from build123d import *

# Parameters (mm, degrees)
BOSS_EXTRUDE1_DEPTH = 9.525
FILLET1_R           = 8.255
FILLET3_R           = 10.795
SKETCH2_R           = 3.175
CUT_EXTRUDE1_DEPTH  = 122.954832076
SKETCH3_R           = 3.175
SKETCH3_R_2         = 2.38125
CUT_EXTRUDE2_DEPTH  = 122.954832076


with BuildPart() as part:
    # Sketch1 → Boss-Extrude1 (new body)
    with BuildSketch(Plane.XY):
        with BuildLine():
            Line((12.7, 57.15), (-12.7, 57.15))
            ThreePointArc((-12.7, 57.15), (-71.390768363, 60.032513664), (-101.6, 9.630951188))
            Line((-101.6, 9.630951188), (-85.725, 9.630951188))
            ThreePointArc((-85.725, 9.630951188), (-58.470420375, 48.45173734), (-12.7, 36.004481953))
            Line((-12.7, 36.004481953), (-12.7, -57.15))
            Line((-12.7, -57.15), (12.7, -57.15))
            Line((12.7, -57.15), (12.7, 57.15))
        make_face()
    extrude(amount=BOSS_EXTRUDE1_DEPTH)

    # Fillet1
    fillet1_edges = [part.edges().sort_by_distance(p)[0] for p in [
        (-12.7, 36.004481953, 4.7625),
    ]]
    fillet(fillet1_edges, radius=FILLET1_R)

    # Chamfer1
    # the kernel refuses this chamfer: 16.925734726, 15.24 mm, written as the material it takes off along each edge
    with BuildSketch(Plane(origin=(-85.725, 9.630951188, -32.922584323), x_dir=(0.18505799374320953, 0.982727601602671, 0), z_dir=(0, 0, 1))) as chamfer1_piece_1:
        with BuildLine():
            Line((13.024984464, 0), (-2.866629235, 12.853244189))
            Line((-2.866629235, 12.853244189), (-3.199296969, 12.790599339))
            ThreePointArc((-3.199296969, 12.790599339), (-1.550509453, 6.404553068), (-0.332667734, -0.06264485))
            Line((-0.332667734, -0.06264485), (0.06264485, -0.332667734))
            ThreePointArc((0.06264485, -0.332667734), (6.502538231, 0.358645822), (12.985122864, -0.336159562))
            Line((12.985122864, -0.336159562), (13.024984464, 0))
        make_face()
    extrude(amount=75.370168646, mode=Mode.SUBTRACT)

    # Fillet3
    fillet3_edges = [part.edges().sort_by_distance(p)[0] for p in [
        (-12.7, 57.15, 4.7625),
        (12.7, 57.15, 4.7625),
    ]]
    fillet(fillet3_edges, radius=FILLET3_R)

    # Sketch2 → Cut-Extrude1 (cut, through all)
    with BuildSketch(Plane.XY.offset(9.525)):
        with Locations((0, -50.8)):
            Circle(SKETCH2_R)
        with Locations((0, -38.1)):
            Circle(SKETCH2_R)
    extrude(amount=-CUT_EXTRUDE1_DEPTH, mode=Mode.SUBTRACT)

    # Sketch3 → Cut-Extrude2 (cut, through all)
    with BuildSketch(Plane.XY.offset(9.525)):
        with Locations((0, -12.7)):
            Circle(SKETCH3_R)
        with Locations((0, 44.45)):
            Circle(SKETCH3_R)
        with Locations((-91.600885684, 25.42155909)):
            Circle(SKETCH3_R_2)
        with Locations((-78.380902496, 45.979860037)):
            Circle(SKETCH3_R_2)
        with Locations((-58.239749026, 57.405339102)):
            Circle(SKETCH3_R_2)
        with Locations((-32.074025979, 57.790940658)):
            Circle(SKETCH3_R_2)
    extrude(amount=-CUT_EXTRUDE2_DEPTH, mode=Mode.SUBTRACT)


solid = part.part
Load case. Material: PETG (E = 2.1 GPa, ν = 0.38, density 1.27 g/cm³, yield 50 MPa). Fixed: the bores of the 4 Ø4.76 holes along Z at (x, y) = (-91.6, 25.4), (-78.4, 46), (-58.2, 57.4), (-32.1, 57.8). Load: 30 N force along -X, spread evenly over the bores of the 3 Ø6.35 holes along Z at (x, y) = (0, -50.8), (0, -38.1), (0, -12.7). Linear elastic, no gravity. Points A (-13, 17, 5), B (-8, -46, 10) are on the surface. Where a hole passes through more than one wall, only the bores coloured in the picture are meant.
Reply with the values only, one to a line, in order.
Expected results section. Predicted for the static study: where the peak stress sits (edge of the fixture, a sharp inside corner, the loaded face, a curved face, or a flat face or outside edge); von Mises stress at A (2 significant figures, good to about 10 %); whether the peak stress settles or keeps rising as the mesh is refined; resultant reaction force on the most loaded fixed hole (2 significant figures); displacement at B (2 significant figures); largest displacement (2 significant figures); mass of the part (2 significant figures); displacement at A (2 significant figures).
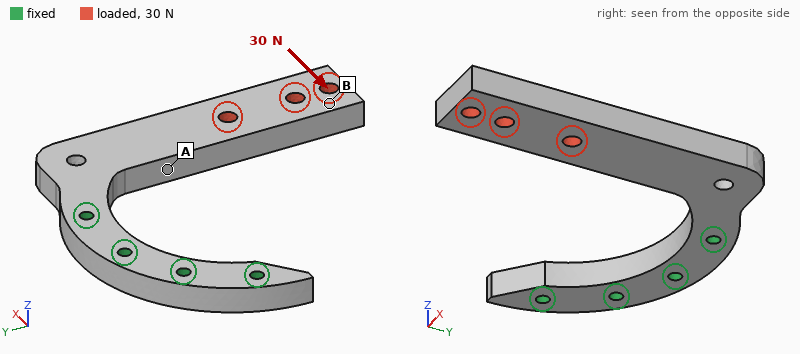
edge of the fixture
1.4 MPa
keeps rising
62 N
1.5 mm
1.7 mm
53 g
0.49 mm
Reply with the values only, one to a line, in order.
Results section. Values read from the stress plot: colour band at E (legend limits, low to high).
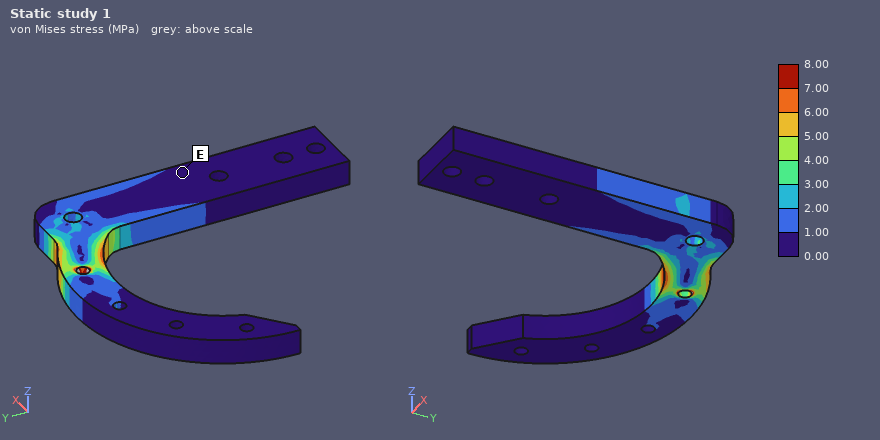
0.00 to 1.00 MPa
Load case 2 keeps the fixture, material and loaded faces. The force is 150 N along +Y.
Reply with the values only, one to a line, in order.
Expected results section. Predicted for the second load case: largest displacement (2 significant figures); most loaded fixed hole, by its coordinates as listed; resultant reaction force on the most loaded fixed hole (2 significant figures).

1.9 mm
(-32.1, 57.8)
250 N
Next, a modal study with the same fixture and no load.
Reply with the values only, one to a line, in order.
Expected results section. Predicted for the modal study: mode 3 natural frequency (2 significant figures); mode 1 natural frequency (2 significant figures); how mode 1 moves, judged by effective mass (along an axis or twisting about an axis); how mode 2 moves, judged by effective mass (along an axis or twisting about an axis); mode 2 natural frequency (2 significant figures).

510 Hz
110 Hz
along Z
along X
180 Hz
